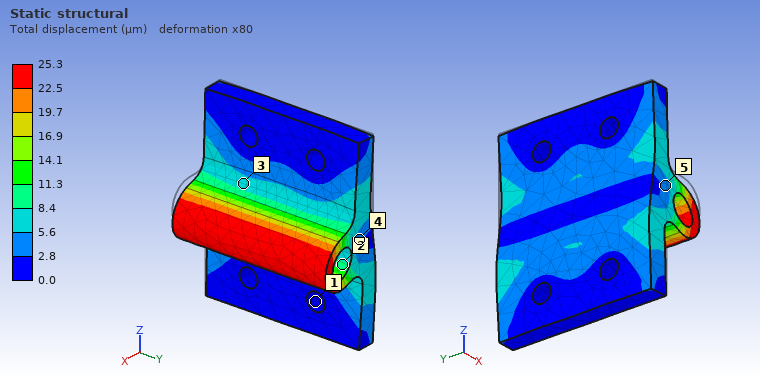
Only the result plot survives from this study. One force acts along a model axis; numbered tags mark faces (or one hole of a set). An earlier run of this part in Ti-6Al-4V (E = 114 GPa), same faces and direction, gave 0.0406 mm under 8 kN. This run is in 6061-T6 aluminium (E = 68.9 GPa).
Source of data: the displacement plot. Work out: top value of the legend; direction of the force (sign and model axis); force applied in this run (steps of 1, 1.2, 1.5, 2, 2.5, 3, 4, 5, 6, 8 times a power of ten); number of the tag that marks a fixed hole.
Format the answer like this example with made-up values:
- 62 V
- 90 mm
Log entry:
- 25.3 µm
- -Z
- 3 kN
- 1
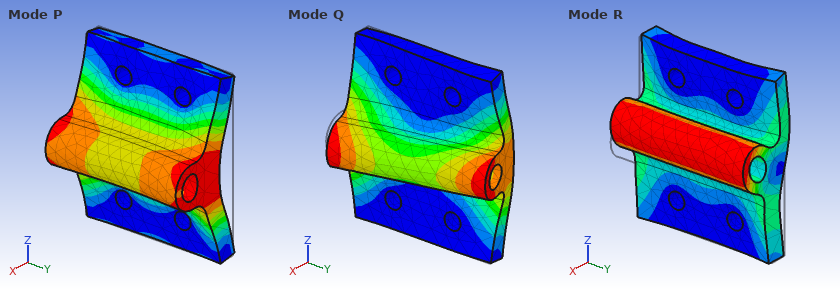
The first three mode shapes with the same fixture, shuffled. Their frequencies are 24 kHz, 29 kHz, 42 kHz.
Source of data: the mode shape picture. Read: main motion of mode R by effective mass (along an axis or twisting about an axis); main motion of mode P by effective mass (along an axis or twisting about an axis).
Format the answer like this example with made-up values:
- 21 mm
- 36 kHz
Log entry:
- along Z
- along X
